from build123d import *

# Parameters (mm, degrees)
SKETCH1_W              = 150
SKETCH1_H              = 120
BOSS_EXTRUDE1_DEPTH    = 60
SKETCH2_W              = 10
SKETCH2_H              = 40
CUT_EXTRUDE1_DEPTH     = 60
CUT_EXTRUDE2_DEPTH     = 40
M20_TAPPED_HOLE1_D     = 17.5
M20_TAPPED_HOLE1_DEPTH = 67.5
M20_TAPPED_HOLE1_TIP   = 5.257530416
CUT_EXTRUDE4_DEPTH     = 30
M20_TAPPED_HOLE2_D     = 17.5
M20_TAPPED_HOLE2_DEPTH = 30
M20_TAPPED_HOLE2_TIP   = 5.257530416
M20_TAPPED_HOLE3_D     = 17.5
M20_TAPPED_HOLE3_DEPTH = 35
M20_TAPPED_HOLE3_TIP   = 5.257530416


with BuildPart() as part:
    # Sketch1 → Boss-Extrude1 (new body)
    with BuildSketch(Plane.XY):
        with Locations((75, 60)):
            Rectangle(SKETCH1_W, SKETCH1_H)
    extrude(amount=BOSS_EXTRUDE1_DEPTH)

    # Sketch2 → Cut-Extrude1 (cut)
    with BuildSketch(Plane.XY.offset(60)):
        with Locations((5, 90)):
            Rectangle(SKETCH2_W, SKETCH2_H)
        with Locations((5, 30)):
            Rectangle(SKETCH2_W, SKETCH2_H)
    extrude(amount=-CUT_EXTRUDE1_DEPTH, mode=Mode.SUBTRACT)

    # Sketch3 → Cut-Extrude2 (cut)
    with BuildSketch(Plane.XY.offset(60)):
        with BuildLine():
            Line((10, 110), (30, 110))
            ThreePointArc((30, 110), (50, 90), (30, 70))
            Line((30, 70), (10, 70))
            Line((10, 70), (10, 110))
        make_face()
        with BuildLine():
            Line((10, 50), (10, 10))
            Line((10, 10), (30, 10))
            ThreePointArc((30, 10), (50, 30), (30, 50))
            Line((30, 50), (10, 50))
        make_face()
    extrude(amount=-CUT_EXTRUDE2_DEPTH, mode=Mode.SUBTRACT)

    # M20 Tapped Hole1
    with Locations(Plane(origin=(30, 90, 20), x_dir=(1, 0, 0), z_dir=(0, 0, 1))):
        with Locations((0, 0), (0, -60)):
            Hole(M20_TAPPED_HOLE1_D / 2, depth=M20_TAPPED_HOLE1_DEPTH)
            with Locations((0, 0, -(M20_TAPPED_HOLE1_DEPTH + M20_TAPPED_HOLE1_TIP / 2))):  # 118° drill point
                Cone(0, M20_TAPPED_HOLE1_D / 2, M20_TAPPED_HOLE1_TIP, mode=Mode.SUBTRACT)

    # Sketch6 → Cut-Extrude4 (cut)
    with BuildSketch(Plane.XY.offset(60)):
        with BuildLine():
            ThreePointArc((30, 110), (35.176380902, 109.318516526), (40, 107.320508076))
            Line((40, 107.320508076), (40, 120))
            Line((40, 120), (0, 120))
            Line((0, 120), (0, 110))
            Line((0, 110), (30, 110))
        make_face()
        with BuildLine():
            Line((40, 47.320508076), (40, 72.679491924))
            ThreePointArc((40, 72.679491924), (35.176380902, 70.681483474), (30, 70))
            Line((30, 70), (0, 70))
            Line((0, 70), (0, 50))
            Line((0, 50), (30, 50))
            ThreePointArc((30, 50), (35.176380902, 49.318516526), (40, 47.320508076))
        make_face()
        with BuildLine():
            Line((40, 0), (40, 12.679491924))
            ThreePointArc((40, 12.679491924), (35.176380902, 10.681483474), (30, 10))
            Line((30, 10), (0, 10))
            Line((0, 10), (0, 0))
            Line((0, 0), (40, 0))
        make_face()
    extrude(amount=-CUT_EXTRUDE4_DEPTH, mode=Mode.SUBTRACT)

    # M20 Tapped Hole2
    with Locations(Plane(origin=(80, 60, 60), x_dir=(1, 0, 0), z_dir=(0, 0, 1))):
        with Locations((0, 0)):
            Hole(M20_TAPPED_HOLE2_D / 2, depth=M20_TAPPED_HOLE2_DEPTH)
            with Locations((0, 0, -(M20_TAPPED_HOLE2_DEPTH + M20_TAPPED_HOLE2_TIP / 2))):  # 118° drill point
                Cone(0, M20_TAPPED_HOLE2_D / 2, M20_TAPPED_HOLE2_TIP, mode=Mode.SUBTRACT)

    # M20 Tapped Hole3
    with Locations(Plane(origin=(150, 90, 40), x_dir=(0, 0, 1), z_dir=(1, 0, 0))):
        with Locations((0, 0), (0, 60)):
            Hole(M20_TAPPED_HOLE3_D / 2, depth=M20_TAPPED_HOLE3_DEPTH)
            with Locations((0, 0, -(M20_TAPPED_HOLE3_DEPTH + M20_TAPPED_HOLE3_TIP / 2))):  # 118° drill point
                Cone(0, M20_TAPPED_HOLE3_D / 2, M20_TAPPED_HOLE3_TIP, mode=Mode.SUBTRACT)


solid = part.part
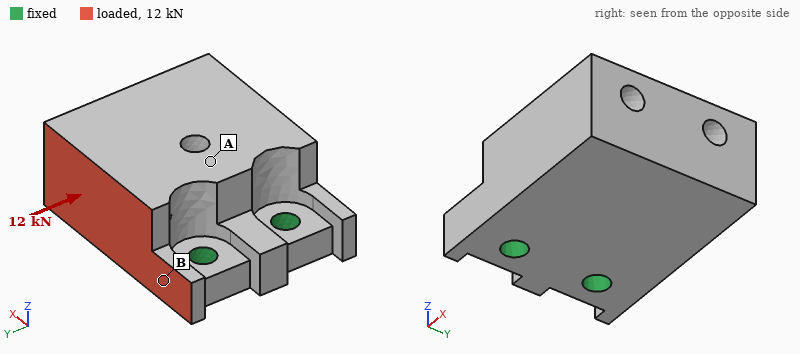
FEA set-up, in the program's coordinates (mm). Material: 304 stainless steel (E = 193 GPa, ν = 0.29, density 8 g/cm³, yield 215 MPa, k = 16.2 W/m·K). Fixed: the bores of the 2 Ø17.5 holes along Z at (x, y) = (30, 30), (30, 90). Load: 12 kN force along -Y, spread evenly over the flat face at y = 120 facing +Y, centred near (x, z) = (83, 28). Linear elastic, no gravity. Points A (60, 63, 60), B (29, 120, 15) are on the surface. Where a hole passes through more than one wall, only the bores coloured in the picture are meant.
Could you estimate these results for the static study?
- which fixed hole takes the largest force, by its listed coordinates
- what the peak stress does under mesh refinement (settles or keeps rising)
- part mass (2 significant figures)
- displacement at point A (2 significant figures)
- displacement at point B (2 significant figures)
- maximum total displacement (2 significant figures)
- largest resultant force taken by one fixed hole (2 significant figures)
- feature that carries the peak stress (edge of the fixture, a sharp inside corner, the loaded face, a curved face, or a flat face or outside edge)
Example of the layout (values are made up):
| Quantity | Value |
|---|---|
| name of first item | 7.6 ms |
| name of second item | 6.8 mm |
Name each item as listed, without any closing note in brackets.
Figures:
| Quantity | Value |
|---|---|
| which fixed hole takes the largest force, by its listed coordinates | (30, 90) |
| what the peak stress does under mesh refinement | keeps rising |
| part mass | 6.7 kg |
| displacement at point A | 3.8 µm |
| displacement at point B | 2.6 µm |
| maximum total displacement | 10.0 µm |
| largest resultant force taken by one fixed hole | 11 kN |
| feature that carries the peak stress | edge of the fixture |
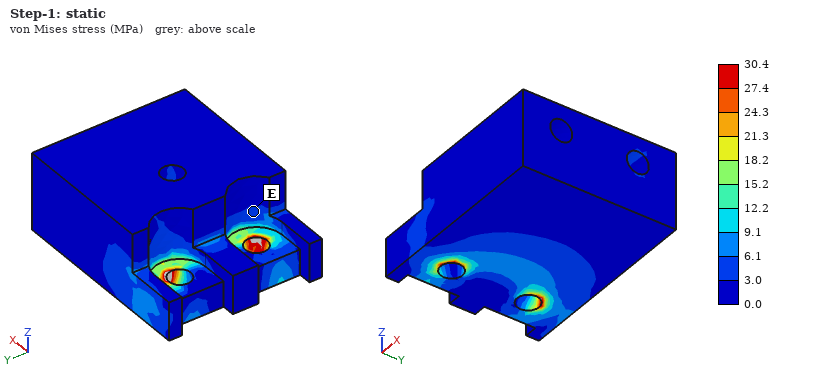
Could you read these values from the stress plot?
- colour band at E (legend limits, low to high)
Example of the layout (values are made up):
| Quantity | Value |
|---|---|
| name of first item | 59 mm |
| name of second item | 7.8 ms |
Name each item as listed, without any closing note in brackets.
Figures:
| Quantity | Value |
|---|---|
| colour band at E | 3.0 to 6.1 MPa |
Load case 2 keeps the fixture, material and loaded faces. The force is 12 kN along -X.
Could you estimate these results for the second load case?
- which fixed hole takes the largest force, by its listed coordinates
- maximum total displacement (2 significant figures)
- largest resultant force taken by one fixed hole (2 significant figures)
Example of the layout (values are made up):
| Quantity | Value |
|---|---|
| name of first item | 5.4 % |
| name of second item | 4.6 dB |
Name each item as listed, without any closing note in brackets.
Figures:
| Quantity | Value |
|---|---|
| which fixed hole takes the largest force, by its listed coordinates | (30, 90) |
| maximum total displacement | 30 µm |
| largest resultant force taken by one fixed hole | 16 kN |
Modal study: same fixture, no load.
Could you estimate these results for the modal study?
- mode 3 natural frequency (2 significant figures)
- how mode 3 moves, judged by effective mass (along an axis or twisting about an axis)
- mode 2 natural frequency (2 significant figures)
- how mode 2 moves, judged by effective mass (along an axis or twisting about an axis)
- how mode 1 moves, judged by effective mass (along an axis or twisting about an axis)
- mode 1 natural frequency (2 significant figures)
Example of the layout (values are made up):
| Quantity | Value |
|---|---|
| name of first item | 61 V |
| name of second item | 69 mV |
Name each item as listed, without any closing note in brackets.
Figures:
| Quantity | Value |
|---|---|
| mode 3 natural frequency | 3100 Hz |
| how mode 3 moves, judged by effective mass | twisting about X |
| mode 2 natural frequency | 2500 Hz |
| how mode 2 moves, judged by effective mass | along Y |
| how mode 1 moves, judged by effective mass | along Z |
| mode 1 natural frequency | 930 Hz |
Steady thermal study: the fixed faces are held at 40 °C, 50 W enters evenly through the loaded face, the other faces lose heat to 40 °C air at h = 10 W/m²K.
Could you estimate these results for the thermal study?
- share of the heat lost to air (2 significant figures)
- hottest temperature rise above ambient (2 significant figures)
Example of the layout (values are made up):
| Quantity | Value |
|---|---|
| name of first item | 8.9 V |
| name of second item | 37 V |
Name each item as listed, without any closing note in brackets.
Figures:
| Quantity | Value |
|---|---|
| share of the heat lost to air | 27 % |
| hottest temperature rise above ambient | 47 K |
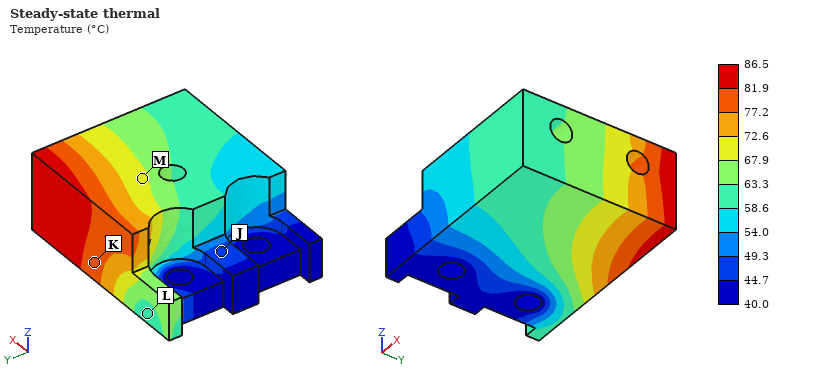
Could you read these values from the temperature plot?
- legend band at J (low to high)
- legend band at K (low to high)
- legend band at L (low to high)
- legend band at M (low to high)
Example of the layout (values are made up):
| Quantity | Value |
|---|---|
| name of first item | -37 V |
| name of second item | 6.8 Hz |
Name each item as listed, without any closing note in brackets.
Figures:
| Quantity | Value |
|---|---|
| legend band at J | 44.7 to 49.3 °C |
| legend band at K | 77.2 to 81.9 °C |
| legend band at L | 58.6 to 63.3 °C |
| legend band at M | 67.9 to 72.6 °C |
